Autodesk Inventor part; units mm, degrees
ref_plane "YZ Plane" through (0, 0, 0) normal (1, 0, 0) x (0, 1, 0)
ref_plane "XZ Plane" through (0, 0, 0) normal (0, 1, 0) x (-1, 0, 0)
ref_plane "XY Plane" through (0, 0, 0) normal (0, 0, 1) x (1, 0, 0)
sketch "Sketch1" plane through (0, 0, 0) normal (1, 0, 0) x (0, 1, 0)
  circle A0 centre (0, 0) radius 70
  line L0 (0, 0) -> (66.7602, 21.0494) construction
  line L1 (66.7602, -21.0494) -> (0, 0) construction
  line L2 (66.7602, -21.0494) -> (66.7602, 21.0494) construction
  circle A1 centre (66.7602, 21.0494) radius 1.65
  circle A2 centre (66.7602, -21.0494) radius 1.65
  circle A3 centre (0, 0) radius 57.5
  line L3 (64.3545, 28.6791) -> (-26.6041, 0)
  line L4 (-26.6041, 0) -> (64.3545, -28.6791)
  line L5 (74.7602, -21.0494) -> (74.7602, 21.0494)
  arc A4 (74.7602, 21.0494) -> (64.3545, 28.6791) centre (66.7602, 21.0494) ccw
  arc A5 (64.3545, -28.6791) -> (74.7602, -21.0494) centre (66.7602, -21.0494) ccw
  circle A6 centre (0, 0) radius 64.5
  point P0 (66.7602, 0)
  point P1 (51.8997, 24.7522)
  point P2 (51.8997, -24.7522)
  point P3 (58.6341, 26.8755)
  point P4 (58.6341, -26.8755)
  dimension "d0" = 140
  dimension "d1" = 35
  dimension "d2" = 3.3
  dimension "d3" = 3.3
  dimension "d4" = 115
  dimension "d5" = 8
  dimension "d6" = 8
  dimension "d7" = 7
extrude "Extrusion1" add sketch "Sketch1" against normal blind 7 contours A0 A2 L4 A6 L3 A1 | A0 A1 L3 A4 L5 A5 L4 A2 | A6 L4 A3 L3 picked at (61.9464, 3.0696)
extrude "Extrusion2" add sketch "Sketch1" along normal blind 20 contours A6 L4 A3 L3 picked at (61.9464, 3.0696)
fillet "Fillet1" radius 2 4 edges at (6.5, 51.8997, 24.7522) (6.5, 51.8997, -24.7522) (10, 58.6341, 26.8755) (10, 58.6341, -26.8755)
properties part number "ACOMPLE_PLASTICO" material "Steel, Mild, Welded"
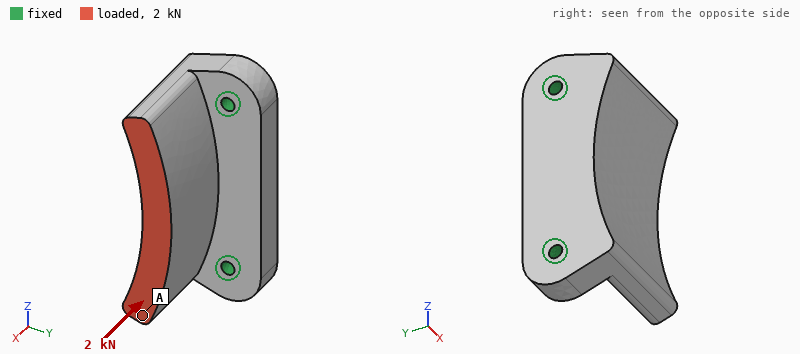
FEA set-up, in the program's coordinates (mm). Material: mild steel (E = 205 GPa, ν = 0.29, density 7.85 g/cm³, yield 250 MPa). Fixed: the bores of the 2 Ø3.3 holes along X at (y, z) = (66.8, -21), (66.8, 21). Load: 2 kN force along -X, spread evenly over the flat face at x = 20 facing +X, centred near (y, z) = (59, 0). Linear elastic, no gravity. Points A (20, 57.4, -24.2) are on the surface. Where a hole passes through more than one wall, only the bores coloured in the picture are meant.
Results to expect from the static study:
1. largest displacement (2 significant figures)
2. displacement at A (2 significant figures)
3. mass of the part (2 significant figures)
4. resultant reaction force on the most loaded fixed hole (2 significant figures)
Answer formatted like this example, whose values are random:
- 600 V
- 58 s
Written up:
- 11 µm
- 9.9 µm
- 110 g
- 1.0 kN
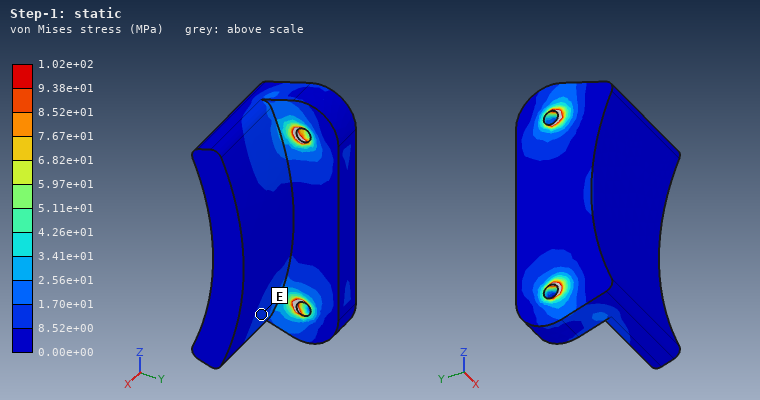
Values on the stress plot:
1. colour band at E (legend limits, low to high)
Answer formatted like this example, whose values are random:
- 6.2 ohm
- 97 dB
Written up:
- 8.52e+00 to 1.70e+01 MPa
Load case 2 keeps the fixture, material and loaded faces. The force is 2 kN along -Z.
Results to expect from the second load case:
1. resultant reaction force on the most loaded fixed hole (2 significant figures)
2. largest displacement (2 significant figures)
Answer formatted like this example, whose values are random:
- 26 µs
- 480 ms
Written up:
- 1.5 kN
- 7.9 µm
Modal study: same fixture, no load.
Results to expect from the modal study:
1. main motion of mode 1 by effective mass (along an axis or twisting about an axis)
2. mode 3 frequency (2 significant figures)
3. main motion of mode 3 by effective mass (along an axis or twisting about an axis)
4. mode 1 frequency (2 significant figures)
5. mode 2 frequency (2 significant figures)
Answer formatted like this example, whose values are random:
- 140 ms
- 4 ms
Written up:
- along Y
- 15 kHz
- along X
- 5900 Hz
- 11 kHz
